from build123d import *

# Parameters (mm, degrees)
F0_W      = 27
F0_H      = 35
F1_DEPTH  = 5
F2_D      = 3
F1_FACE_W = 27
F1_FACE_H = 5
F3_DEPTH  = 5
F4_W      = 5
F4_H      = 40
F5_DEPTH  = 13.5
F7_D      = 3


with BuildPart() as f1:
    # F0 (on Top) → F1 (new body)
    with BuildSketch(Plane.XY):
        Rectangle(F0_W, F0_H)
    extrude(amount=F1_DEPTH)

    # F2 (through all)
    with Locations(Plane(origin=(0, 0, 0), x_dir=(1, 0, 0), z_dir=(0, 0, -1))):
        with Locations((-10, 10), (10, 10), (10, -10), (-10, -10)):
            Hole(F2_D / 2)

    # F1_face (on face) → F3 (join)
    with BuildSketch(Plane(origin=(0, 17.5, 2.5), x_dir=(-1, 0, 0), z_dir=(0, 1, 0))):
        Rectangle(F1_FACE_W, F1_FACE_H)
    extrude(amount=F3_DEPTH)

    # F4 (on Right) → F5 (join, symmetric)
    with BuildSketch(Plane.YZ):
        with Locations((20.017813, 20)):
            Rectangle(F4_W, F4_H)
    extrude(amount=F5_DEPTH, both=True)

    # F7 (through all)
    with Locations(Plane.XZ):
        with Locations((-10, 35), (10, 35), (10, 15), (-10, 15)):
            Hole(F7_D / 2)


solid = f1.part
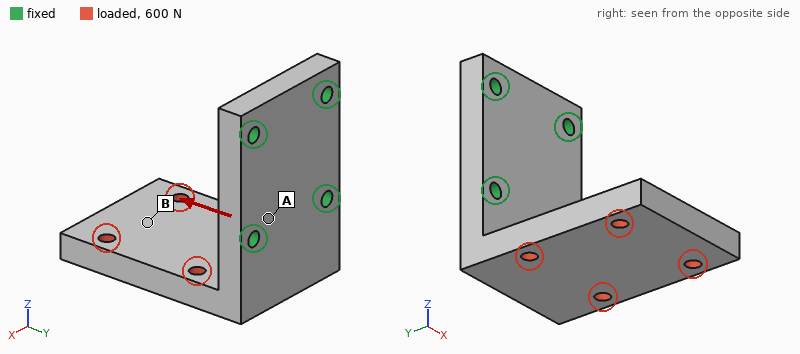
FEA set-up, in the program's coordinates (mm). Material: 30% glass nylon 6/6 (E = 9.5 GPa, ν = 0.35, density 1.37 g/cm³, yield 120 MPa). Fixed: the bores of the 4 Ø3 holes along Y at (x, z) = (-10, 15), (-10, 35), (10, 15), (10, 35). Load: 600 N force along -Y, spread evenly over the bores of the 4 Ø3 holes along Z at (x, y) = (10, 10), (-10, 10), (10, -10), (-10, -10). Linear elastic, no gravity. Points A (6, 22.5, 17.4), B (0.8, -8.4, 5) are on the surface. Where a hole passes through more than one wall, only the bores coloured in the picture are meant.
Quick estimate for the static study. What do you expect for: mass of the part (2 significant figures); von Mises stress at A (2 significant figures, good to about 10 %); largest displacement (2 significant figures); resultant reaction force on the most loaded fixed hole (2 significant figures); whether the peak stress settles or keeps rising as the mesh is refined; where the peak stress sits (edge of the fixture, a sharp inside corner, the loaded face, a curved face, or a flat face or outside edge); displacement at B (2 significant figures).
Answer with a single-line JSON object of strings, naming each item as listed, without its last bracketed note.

{"mass of the part": "13 g", "von Mises stress at A": "19 MPa", "largest displacement": "0.73 mm", "resultant reaction force on the most loaded fixed hole": "350 N", "whether the peak stress settles or keeps rising as the mesh is refined": "keeps rising", "where the peak stress sits": "edge of the fixture", "displacement at B": "0.54 mm"}
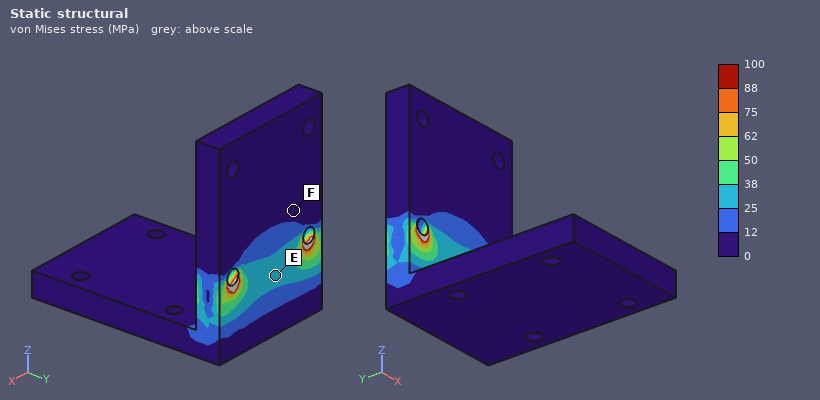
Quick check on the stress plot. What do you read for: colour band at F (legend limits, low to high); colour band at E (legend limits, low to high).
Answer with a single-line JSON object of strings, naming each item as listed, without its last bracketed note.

{"colour band at F": "0 to 12 MPa", "colour band at E": "25 to 38 MPa"}
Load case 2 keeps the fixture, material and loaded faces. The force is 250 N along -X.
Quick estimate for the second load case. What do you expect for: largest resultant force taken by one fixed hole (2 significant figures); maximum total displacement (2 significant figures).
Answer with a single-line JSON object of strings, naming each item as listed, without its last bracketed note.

{"largest resultant force taken by one fixed hole": "310 N", "maximum total displacement": "0.30 mm"}
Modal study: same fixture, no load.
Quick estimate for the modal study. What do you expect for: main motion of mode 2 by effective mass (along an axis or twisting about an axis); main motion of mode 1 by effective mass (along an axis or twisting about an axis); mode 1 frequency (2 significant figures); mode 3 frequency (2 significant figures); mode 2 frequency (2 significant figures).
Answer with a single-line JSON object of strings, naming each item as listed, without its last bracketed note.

{"main motion of mode 2 by effective mass": "along X", "main motion of mode 1 by effective mass": "along Z", "mode 1 frequency": "1000 Hz", "mode 3 frequency": "4200 Hz", "mode 2 frequency": "2200 Hz"}
